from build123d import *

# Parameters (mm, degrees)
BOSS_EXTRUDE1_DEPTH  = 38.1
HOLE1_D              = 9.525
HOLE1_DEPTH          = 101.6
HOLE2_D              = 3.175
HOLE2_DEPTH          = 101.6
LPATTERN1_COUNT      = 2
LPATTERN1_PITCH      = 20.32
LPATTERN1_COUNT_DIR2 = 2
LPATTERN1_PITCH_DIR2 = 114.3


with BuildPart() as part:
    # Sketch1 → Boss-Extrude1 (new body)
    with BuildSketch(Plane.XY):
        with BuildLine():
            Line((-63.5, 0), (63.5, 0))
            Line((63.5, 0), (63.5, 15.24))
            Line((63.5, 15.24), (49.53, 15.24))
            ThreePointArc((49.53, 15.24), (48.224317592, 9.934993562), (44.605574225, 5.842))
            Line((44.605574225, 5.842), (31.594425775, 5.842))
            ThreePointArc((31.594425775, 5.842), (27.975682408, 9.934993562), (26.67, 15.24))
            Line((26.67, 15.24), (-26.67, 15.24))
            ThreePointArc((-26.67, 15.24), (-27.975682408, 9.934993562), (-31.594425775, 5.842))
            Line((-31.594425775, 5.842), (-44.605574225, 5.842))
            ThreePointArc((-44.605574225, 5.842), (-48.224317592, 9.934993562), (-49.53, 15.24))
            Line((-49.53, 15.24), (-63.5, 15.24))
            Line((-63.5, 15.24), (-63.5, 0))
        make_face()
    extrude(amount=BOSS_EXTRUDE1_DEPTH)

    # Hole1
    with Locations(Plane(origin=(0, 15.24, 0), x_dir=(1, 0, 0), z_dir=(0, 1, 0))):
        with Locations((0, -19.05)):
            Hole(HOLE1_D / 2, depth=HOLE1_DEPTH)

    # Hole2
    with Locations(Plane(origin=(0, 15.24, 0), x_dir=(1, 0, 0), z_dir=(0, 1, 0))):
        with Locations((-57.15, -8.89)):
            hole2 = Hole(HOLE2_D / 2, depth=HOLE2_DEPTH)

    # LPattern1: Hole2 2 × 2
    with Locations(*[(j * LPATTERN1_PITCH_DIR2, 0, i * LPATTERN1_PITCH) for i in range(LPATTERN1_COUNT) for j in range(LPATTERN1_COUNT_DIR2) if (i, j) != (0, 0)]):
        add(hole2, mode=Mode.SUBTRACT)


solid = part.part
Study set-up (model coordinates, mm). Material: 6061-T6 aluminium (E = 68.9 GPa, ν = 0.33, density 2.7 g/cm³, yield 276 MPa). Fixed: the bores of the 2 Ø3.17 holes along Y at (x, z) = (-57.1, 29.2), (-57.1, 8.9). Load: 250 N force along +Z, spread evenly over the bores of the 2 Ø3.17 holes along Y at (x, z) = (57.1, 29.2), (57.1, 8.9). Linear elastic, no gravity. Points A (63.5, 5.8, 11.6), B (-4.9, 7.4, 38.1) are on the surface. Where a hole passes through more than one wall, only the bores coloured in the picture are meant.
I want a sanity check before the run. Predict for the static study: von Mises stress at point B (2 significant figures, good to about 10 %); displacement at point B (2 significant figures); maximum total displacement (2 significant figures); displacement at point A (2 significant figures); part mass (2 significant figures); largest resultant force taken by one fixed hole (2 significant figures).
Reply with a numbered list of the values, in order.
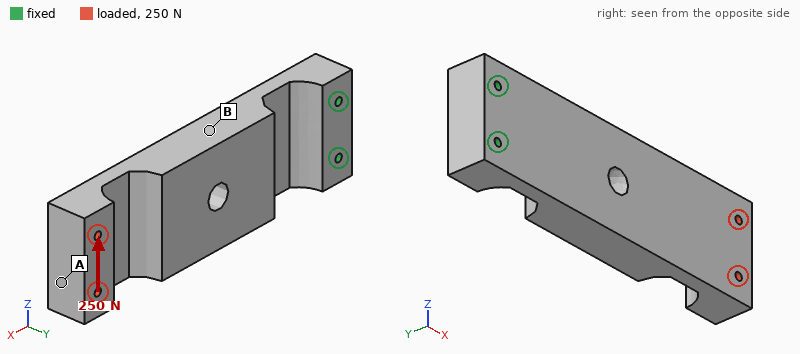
1. 4.5 MPa
2. 24 µm
3. 72 µm
4. 68 µm
5. 160 g
6. 1.3 kN
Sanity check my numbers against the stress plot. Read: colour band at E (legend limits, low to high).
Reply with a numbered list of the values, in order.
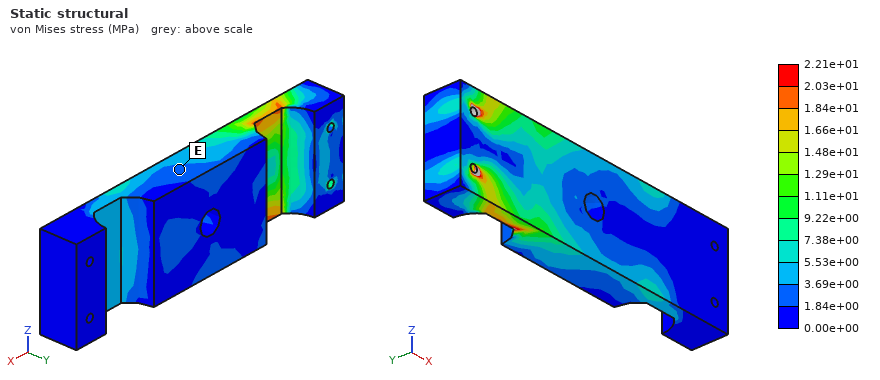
1. 1.84e+00 to 3.69e+00 MPa
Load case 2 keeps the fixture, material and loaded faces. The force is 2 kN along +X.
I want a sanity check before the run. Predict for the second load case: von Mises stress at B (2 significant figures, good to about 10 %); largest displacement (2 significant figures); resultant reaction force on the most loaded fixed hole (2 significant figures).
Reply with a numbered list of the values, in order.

1. 3.6 MPa
2. 0.51 mm
3. 1.0 kN
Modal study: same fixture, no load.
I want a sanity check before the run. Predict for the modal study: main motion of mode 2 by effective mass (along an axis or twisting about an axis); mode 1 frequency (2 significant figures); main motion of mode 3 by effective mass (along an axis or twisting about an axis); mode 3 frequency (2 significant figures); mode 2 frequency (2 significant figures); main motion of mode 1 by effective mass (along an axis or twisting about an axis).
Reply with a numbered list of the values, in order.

1. along Z
2. 350 Hz
3. twisting about X
4. 2700 Hz
5. 1500 Hz
6. along Y
